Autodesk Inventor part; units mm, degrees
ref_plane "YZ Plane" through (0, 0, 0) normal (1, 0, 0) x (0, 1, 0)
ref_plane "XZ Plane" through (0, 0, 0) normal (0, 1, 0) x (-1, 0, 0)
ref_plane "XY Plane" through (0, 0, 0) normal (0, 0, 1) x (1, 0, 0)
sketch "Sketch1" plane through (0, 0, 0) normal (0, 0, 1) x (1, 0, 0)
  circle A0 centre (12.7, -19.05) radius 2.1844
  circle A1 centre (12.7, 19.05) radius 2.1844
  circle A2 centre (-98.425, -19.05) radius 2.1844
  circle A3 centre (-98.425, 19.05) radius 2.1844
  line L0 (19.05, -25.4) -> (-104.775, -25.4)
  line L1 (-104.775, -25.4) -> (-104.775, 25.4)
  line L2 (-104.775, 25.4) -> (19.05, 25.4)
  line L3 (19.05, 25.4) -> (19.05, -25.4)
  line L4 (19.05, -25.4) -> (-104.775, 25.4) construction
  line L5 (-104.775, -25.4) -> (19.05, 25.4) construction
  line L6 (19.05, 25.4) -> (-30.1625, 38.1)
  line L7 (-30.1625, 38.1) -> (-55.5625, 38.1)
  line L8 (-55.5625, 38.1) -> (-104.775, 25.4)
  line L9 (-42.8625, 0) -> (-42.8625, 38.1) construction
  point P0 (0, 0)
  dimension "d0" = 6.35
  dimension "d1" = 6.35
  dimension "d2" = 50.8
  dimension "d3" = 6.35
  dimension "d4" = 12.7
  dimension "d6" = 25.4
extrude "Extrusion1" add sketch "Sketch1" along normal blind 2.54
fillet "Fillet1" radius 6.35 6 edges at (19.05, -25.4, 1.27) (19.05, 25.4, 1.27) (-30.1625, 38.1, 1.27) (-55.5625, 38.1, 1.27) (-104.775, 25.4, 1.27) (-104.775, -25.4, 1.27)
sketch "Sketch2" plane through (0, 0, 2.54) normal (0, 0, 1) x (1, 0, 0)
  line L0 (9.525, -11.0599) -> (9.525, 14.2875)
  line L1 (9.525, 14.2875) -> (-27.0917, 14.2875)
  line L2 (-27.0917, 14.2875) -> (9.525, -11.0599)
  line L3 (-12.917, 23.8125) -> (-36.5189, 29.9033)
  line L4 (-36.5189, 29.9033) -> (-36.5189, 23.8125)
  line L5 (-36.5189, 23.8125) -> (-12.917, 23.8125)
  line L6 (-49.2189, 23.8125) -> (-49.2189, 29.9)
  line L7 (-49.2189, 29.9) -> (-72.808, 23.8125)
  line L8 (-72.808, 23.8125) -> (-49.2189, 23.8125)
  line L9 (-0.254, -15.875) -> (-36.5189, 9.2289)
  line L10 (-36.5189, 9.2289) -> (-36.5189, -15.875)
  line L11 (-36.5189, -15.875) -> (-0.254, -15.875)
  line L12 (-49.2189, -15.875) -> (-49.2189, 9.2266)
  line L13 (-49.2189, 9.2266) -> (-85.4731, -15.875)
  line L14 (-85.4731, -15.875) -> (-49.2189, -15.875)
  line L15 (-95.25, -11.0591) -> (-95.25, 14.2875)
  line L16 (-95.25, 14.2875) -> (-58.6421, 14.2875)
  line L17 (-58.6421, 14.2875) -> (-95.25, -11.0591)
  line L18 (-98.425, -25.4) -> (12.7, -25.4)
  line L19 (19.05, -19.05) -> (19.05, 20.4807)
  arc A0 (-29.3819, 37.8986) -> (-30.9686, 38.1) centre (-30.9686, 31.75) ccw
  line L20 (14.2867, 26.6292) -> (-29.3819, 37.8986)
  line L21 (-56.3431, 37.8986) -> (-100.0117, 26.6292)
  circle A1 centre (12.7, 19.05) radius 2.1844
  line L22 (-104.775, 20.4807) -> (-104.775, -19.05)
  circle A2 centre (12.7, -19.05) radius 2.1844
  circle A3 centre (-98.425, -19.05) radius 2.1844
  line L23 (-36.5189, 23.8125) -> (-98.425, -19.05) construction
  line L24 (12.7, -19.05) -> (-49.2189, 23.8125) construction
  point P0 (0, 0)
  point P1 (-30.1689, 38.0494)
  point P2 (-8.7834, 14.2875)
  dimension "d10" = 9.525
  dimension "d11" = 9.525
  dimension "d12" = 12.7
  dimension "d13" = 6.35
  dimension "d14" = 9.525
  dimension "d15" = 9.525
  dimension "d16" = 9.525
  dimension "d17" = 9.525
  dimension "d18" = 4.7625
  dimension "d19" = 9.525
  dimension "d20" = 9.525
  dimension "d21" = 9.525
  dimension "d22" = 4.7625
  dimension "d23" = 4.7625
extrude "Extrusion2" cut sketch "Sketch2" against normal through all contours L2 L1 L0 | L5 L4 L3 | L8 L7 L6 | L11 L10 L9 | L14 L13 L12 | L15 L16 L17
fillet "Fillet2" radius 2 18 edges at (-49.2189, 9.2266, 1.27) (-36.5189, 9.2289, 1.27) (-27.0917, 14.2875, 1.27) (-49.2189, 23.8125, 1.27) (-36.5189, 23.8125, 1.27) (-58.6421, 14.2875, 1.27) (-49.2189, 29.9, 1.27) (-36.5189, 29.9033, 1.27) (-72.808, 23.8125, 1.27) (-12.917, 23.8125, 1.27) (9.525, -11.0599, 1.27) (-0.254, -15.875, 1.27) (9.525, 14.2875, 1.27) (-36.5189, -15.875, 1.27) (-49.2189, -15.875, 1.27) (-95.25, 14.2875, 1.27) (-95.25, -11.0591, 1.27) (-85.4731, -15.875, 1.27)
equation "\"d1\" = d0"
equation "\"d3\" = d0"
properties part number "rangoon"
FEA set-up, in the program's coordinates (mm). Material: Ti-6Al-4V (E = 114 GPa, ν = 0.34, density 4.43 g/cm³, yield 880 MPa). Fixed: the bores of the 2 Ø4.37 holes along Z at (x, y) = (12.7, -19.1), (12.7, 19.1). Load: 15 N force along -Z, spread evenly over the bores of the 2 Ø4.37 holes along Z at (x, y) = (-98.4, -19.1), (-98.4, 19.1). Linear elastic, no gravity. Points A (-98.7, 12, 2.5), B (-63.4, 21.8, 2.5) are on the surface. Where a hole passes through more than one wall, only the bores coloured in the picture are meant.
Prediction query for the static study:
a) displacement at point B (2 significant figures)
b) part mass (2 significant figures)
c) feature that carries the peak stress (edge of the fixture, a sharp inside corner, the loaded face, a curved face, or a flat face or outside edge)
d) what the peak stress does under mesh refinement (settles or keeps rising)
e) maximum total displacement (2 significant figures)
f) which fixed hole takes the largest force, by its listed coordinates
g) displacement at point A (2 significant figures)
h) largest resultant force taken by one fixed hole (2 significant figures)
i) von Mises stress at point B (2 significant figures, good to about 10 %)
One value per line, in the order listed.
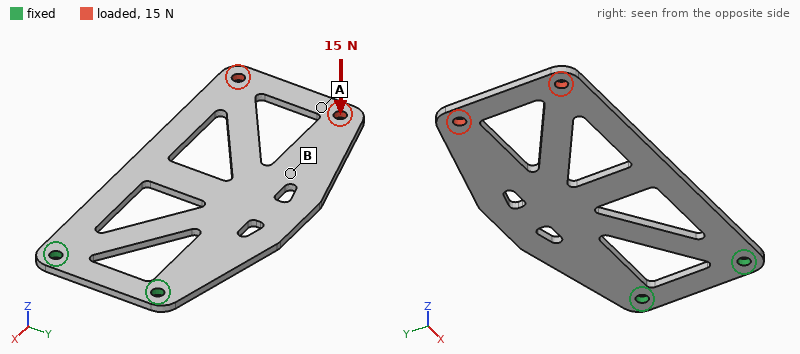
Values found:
0.65 mm
59 g
edge of the fixture
keeps rising
1.3 mm
(12.7, -19.1)
1.2 mm
9.5 N
11 MPa
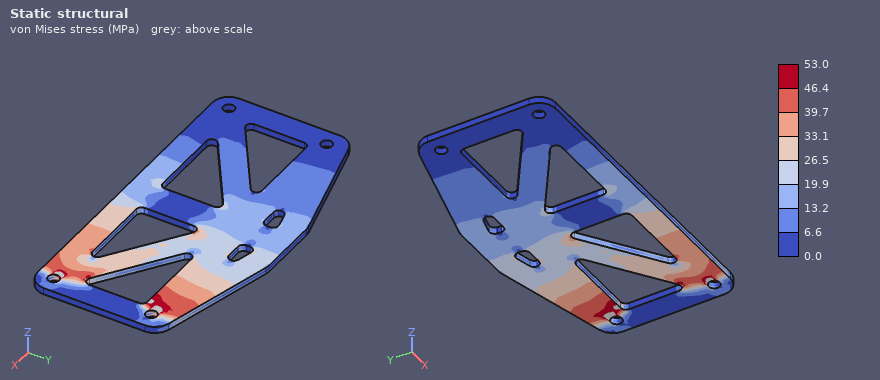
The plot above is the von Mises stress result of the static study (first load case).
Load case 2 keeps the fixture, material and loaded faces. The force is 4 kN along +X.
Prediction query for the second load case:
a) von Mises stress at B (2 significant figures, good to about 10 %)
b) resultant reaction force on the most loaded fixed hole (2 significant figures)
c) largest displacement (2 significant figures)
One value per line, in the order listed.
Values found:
38 MPa
2.1 kN
81 µm
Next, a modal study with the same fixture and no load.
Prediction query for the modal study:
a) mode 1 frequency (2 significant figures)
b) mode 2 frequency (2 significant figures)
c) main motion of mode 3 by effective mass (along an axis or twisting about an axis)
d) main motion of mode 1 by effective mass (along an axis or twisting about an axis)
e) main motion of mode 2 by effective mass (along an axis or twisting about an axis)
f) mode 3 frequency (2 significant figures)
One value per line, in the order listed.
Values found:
140 Hz
550 Hz
along Z
along Z
twisting about X
870 Hz
